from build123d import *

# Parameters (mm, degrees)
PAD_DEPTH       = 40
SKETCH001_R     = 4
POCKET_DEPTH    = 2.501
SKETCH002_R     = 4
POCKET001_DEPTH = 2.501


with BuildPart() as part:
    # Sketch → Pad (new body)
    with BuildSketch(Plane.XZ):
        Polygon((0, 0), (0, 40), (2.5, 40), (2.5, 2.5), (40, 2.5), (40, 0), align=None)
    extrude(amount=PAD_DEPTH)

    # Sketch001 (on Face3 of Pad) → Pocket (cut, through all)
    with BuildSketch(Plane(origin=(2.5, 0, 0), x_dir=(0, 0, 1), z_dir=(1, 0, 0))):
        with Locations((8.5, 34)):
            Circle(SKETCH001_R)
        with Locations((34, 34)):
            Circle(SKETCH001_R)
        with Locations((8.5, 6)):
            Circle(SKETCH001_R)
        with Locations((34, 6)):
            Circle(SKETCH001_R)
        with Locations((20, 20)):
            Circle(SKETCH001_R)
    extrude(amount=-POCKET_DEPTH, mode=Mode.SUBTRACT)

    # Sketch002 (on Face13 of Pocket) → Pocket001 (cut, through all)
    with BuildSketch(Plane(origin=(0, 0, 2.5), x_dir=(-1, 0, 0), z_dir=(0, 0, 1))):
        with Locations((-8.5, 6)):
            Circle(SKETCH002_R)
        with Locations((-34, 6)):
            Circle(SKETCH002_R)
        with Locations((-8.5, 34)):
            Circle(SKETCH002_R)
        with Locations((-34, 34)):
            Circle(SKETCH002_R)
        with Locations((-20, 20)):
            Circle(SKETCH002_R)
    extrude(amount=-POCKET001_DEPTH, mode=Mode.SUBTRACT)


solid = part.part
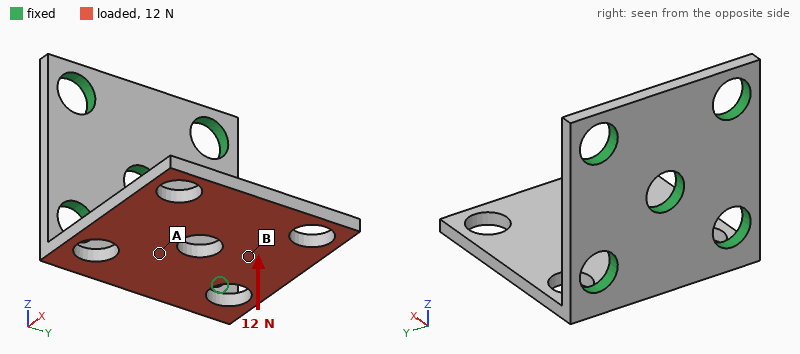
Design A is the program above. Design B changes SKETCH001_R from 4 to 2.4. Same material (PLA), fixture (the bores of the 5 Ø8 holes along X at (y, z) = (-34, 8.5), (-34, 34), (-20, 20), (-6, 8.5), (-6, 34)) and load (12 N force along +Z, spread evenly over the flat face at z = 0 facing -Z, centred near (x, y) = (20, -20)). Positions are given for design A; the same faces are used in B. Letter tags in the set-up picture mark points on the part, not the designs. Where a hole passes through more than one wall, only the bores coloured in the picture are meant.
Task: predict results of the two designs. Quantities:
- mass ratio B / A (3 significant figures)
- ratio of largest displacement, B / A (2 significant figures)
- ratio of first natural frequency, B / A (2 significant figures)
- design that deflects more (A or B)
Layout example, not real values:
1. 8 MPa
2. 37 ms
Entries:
1. 1.06
2. 1.1
3. 0.95
4. B
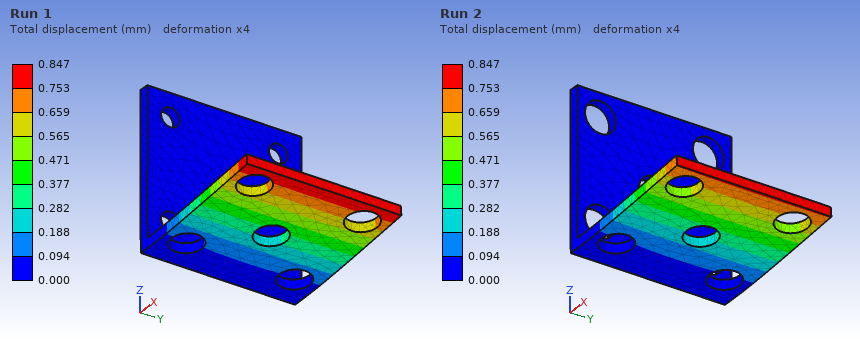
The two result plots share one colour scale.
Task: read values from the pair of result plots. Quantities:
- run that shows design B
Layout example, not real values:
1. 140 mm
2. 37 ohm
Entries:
1. Run 1
